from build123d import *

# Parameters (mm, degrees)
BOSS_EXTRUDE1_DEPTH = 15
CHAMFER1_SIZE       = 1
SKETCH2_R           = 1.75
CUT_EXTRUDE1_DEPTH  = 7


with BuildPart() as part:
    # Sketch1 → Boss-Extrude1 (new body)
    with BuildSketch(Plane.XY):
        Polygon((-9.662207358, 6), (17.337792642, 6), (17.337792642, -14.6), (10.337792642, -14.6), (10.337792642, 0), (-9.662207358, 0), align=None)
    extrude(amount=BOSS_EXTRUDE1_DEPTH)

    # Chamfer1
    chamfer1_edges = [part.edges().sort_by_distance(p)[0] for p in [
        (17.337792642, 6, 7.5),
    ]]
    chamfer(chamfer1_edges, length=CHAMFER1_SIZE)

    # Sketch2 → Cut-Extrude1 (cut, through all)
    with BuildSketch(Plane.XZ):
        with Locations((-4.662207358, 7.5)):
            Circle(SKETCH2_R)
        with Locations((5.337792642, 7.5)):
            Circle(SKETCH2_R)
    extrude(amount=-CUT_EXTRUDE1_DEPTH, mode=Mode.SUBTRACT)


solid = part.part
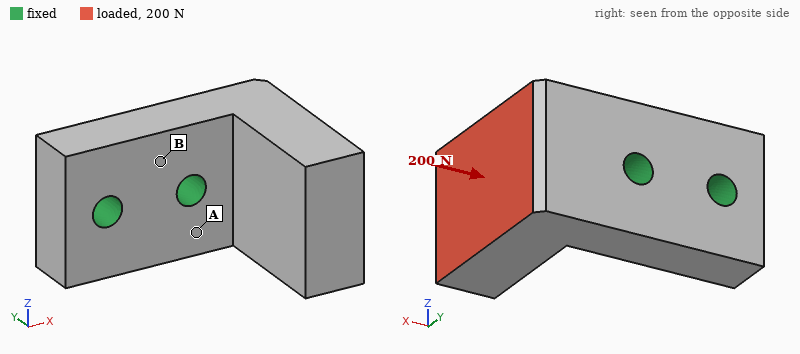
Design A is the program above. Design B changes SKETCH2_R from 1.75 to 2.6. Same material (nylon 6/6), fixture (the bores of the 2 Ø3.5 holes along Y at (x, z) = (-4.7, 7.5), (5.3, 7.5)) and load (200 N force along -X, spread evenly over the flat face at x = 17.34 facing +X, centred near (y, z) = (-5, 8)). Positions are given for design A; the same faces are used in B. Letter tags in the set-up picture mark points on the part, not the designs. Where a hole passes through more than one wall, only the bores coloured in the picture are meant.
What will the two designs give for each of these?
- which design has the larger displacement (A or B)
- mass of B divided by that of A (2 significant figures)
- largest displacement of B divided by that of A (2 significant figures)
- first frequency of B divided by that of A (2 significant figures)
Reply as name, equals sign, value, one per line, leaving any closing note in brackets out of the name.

which design has the larger displacement = A
mass of B divided by that of A = 0.96
largest displacement of B divided by that of A = 0.86
first frequency of B divided by that of A = 1.1
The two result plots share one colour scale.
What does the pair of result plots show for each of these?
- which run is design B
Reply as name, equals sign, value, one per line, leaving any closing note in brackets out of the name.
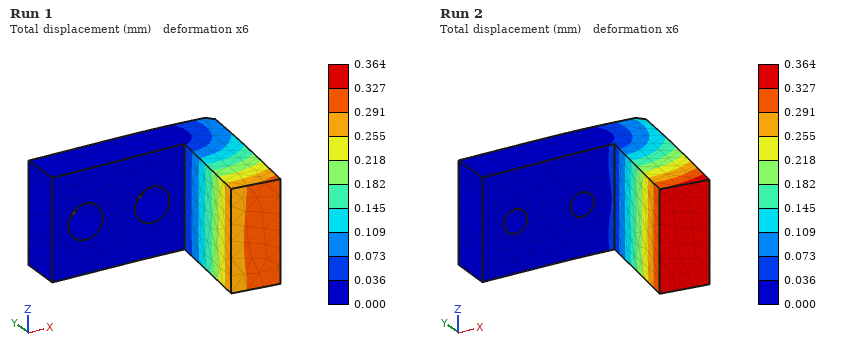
which run is design B = Run 1
